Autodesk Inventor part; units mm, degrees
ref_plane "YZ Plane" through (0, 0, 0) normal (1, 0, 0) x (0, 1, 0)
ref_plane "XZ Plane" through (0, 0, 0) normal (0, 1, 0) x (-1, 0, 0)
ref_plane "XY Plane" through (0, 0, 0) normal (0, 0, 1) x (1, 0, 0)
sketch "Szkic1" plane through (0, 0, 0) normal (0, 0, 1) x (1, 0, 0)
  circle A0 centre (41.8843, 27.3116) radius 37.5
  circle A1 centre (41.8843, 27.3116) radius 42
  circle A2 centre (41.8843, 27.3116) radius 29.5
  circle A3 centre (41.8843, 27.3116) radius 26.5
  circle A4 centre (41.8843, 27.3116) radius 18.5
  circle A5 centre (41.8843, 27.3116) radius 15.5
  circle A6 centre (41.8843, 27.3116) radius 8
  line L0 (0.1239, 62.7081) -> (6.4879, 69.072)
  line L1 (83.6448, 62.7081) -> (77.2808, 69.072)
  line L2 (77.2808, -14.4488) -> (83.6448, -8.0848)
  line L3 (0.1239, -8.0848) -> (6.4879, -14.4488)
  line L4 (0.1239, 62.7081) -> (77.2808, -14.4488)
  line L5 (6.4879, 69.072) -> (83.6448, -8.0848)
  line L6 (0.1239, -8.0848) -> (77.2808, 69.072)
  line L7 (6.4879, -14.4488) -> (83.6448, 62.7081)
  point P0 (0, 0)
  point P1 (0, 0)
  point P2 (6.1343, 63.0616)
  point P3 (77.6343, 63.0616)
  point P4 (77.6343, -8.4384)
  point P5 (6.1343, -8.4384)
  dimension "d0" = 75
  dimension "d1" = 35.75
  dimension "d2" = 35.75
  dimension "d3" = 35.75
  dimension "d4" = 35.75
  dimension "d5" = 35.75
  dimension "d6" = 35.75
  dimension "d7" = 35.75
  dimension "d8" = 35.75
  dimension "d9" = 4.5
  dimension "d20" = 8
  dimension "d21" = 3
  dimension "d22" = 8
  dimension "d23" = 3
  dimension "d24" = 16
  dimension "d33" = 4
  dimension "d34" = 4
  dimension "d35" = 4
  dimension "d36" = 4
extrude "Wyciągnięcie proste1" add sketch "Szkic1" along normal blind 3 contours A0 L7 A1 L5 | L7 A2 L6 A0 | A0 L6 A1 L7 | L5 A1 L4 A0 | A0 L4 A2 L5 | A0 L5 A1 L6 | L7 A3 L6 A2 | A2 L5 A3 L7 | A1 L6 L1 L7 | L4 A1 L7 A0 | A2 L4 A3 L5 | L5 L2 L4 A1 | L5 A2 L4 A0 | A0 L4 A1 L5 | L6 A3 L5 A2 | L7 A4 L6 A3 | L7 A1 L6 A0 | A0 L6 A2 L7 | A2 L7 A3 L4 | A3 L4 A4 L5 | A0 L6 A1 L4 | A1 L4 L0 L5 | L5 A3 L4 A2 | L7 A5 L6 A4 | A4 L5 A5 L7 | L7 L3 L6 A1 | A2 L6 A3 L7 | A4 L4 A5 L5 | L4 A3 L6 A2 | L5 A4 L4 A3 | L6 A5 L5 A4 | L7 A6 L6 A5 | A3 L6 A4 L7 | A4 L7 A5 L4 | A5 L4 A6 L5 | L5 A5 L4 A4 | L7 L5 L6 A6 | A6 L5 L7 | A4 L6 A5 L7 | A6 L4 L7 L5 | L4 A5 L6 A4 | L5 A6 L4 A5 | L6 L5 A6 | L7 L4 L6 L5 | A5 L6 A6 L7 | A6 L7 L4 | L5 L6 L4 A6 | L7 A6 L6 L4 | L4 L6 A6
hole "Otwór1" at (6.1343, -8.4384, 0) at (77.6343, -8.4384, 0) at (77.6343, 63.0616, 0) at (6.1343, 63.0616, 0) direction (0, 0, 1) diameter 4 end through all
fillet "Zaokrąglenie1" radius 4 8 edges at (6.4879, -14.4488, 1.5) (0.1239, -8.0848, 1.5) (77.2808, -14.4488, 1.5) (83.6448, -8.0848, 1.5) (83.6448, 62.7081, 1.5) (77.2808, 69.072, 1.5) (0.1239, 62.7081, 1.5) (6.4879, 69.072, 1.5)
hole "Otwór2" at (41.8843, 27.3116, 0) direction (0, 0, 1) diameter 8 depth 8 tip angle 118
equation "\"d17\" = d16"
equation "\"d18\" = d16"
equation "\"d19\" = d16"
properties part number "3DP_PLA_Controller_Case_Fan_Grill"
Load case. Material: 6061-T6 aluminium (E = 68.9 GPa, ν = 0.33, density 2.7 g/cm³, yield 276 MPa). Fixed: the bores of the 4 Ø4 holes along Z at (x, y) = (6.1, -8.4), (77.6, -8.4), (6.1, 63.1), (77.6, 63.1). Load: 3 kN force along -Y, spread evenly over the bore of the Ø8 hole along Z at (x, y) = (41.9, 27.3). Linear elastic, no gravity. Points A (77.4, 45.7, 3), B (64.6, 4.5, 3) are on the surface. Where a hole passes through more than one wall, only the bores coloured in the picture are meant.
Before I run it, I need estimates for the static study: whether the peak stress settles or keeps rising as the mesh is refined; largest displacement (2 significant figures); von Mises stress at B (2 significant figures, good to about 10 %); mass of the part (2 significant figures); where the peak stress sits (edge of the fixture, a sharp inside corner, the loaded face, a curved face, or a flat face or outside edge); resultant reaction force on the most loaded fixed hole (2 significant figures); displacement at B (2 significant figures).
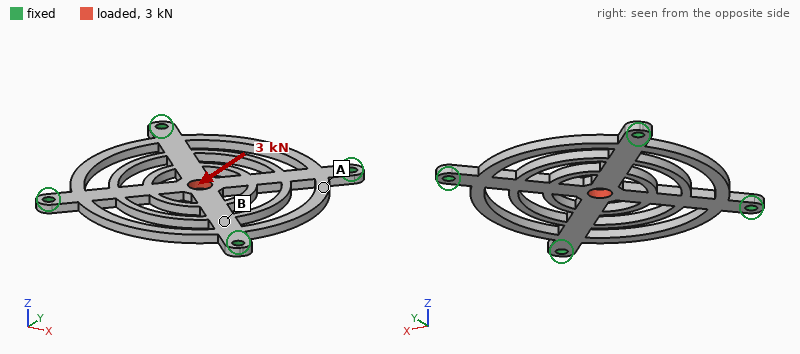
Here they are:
keeps rising
39 µm
37 MPa
27 g
edge of the fixture
1.0 kN
13 µm
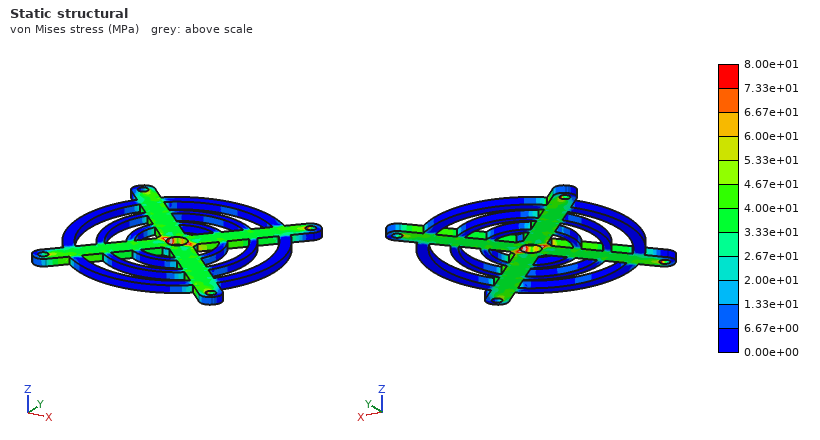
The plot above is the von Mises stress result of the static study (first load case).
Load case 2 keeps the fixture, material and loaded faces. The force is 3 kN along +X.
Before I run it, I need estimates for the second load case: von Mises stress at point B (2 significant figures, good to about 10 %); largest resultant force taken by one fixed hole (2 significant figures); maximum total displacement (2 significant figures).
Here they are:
37 MPa
1.0 kN
38 µm
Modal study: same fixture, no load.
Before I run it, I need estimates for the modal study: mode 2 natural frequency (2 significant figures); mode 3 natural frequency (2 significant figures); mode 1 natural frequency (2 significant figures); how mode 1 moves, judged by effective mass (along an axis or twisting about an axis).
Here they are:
3100 Hz
3100 Hz
1700 Hz
along Z
